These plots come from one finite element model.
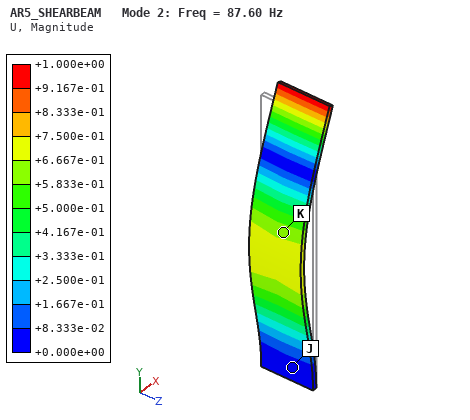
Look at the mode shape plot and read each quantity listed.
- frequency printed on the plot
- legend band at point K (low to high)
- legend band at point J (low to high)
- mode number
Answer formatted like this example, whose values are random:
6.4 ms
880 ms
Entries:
87.60 Hz
+5.833e-01 to +6.667e-01
+0.000e+00 to +8.333e-02
2
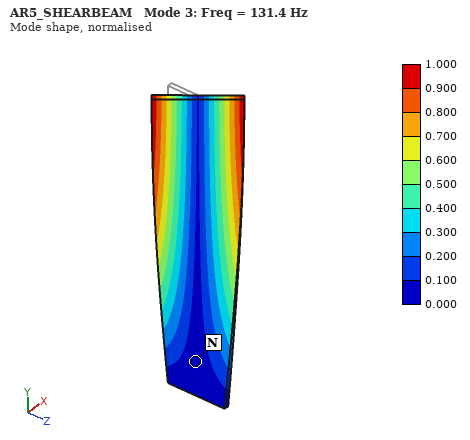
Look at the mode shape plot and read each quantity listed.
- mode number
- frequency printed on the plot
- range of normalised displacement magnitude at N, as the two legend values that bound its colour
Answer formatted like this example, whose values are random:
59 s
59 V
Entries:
3
131.4 Hz
0.000 to 0.100
